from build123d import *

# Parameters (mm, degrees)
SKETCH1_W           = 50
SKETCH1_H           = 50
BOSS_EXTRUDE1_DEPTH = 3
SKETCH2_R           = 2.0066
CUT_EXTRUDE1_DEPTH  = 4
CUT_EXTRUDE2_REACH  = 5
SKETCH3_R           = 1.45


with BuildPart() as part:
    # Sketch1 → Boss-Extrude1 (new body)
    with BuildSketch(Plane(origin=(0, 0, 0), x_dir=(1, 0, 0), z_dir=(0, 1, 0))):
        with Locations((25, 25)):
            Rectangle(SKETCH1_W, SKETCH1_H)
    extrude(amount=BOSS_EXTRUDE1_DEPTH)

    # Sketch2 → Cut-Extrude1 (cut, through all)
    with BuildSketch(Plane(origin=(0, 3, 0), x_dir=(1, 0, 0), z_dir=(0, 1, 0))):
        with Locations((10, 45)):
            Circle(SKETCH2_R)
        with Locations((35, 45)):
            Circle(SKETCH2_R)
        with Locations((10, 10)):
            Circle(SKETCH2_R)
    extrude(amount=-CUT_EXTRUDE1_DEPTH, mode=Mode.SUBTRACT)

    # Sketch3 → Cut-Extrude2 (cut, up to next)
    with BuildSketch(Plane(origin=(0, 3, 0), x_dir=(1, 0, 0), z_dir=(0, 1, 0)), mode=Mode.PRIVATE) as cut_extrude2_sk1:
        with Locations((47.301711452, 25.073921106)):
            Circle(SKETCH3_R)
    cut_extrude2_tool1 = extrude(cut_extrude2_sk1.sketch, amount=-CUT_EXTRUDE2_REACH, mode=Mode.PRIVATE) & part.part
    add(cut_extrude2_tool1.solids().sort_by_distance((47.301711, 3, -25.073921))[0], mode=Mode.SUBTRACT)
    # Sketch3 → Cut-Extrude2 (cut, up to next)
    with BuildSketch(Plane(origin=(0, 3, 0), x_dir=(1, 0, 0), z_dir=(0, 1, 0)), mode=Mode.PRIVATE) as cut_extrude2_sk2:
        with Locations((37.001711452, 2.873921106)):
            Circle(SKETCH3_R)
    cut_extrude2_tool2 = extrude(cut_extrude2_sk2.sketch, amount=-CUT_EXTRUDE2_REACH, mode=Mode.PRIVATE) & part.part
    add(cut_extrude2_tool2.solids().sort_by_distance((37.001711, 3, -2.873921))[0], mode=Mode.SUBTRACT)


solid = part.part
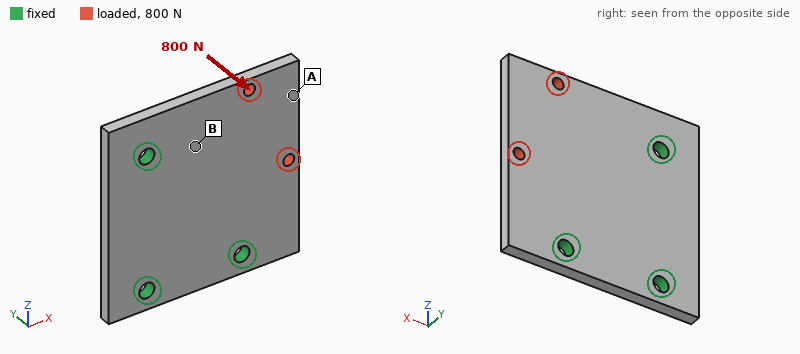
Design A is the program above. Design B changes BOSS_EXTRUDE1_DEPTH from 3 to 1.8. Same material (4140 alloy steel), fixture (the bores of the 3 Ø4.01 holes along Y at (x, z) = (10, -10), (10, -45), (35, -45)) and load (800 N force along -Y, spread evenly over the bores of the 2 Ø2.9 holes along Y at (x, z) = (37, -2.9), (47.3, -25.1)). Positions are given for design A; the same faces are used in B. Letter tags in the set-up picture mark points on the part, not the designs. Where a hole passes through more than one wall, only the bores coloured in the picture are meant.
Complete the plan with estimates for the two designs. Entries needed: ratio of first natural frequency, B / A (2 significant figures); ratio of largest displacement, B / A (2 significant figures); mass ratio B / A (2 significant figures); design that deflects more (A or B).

0.62
4.4
0.60
B
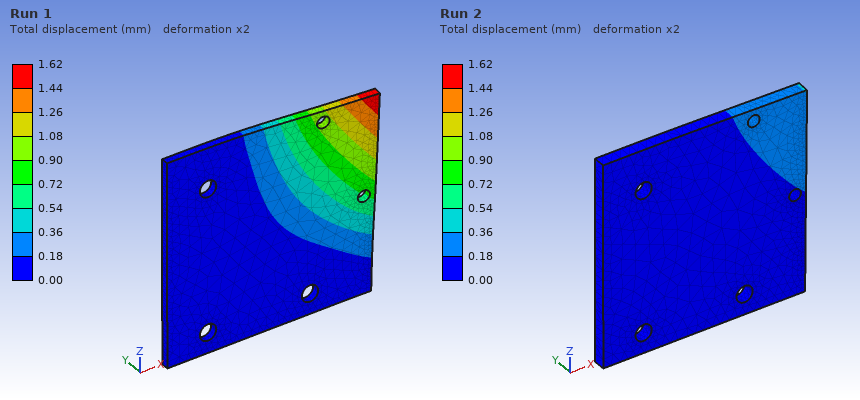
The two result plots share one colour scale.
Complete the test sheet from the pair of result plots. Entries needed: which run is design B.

Run 1
